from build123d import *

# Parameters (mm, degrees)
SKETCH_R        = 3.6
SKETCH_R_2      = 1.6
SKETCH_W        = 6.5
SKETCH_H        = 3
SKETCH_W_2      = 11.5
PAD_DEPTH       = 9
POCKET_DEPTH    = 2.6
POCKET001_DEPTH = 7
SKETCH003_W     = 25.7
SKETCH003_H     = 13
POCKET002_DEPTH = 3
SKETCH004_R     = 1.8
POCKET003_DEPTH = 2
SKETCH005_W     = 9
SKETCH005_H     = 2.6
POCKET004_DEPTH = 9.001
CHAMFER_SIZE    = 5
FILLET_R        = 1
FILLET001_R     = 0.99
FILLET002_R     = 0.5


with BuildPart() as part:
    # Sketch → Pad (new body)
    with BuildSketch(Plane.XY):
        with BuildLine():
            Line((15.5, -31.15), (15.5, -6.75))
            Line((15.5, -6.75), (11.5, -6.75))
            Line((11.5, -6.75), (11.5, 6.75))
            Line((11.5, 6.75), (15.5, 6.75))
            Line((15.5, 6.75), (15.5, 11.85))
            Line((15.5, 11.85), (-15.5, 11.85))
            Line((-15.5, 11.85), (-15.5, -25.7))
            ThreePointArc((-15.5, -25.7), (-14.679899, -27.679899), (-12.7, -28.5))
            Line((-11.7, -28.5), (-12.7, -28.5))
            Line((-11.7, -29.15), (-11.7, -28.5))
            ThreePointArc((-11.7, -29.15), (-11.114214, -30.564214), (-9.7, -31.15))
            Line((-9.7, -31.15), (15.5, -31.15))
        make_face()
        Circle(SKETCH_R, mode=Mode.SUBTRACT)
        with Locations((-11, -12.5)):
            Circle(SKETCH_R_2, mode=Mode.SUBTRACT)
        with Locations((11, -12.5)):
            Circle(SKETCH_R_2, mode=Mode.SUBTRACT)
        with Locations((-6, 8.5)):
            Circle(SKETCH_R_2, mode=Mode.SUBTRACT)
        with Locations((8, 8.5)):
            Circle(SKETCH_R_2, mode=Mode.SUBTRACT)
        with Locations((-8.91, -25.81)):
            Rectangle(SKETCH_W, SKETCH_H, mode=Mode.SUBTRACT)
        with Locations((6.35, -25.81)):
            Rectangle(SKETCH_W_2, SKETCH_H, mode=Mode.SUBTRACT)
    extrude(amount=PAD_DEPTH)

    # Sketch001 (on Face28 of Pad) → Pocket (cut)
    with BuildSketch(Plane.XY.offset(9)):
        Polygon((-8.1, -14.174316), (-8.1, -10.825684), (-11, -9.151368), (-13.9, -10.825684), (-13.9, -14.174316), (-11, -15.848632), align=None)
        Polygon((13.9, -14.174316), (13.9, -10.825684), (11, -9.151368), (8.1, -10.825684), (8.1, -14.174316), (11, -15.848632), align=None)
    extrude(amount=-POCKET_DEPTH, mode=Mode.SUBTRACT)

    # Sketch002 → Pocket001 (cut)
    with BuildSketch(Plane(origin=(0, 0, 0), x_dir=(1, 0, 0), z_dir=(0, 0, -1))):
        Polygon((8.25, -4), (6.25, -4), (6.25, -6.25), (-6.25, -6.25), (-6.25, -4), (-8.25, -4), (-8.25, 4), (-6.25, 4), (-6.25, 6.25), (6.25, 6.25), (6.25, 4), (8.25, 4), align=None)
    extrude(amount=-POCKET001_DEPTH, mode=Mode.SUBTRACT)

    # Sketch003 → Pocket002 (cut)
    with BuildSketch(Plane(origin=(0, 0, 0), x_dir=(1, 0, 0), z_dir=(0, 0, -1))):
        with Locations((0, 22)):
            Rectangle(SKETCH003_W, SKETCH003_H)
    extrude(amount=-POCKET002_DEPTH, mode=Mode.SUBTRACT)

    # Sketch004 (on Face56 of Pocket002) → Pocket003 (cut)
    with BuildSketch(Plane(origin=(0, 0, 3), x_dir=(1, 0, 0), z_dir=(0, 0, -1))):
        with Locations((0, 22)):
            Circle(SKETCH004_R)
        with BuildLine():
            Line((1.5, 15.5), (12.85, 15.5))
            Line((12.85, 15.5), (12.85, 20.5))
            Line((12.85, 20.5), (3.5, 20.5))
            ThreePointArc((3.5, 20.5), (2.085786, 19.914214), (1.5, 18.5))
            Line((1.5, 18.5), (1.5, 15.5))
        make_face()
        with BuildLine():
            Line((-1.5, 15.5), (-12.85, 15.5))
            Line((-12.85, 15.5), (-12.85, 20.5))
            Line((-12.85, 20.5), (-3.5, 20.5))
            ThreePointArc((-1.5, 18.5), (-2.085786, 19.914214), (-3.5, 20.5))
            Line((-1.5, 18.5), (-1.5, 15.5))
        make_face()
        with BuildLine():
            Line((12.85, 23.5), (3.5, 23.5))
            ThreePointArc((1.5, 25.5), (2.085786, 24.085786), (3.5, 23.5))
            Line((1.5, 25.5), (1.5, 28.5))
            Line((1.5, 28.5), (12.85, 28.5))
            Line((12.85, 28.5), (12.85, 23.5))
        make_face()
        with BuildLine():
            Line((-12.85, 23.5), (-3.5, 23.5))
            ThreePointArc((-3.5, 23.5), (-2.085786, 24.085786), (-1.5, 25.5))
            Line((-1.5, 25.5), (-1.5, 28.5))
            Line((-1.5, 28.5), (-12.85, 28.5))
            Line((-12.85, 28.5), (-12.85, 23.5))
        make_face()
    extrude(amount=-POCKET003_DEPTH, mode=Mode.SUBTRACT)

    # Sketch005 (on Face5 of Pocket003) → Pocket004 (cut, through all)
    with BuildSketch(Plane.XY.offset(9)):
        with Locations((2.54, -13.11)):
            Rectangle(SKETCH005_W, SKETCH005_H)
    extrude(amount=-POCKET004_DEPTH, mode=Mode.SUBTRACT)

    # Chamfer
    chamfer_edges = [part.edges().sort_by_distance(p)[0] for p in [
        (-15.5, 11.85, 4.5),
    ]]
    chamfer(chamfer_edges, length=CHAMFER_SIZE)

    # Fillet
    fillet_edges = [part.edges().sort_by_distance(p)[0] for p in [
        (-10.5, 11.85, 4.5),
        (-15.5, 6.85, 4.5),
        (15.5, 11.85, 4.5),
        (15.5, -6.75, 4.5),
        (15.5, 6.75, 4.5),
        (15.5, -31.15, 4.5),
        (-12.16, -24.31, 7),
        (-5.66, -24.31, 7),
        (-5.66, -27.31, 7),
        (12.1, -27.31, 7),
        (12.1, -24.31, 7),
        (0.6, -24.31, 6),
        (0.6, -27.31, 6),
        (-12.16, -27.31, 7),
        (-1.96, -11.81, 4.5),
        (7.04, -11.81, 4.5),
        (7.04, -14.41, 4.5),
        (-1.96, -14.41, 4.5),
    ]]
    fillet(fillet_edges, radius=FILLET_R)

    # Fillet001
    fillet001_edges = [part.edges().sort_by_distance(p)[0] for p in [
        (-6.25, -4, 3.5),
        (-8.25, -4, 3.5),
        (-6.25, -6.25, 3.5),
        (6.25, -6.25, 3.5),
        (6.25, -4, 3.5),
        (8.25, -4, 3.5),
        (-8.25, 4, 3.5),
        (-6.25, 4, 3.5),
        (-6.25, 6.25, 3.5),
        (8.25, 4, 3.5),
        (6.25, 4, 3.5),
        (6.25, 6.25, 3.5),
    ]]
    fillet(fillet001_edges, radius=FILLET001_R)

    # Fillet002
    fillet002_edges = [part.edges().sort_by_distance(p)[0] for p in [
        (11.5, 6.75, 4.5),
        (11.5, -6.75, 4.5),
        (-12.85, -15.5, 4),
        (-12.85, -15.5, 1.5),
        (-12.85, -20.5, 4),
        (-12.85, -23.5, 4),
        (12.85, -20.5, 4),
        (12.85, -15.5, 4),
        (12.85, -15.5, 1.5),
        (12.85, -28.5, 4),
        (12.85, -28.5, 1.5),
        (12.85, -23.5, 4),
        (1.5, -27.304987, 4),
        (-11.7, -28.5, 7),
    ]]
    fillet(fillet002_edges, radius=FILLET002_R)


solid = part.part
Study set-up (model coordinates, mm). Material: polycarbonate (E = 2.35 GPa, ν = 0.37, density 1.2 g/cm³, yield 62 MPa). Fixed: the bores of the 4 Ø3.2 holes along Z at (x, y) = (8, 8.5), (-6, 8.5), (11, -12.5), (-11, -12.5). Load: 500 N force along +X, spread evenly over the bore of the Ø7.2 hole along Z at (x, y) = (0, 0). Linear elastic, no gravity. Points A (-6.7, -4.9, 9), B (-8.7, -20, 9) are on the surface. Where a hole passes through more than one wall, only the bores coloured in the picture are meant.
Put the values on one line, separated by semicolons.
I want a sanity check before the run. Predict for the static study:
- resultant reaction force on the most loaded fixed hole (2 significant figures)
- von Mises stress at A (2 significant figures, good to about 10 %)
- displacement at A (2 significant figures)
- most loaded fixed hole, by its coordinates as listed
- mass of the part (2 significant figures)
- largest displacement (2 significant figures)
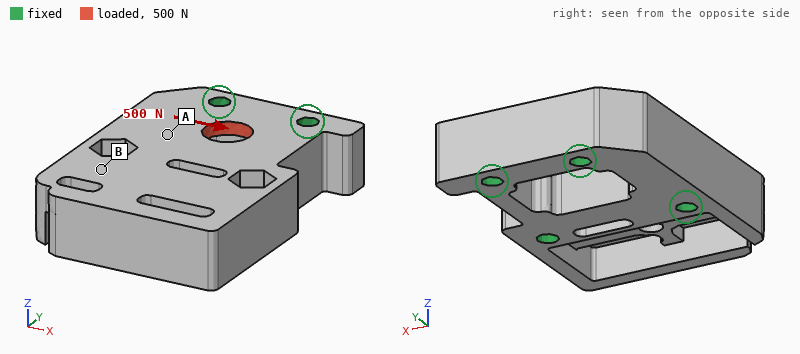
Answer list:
160 N; 6.3 MPa; 24 µm; (-6, 8.5); 9.1 g; 51 µm
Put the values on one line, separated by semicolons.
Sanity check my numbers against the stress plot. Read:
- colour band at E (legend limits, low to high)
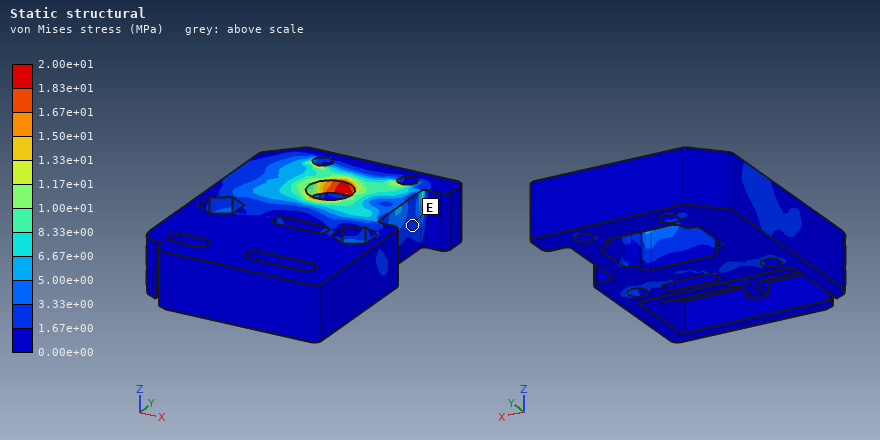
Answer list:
1.67e+00 to 3.33e+00 MPa
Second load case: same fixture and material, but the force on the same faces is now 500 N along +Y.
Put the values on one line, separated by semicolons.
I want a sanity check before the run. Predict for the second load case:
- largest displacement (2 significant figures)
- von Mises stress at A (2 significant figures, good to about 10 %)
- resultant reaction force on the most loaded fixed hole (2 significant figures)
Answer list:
55 µm; 4.9 MPa; 180 N
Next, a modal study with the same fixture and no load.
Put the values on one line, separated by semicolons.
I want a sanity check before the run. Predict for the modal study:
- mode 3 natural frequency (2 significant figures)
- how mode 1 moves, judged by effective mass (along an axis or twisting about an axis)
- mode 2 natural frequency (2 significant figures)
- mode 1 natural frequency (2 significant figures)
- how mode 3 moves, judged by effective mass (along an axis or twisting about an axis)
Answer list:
7000 Hz; along Z; 4400 Hz; 2700 Hz; along X
